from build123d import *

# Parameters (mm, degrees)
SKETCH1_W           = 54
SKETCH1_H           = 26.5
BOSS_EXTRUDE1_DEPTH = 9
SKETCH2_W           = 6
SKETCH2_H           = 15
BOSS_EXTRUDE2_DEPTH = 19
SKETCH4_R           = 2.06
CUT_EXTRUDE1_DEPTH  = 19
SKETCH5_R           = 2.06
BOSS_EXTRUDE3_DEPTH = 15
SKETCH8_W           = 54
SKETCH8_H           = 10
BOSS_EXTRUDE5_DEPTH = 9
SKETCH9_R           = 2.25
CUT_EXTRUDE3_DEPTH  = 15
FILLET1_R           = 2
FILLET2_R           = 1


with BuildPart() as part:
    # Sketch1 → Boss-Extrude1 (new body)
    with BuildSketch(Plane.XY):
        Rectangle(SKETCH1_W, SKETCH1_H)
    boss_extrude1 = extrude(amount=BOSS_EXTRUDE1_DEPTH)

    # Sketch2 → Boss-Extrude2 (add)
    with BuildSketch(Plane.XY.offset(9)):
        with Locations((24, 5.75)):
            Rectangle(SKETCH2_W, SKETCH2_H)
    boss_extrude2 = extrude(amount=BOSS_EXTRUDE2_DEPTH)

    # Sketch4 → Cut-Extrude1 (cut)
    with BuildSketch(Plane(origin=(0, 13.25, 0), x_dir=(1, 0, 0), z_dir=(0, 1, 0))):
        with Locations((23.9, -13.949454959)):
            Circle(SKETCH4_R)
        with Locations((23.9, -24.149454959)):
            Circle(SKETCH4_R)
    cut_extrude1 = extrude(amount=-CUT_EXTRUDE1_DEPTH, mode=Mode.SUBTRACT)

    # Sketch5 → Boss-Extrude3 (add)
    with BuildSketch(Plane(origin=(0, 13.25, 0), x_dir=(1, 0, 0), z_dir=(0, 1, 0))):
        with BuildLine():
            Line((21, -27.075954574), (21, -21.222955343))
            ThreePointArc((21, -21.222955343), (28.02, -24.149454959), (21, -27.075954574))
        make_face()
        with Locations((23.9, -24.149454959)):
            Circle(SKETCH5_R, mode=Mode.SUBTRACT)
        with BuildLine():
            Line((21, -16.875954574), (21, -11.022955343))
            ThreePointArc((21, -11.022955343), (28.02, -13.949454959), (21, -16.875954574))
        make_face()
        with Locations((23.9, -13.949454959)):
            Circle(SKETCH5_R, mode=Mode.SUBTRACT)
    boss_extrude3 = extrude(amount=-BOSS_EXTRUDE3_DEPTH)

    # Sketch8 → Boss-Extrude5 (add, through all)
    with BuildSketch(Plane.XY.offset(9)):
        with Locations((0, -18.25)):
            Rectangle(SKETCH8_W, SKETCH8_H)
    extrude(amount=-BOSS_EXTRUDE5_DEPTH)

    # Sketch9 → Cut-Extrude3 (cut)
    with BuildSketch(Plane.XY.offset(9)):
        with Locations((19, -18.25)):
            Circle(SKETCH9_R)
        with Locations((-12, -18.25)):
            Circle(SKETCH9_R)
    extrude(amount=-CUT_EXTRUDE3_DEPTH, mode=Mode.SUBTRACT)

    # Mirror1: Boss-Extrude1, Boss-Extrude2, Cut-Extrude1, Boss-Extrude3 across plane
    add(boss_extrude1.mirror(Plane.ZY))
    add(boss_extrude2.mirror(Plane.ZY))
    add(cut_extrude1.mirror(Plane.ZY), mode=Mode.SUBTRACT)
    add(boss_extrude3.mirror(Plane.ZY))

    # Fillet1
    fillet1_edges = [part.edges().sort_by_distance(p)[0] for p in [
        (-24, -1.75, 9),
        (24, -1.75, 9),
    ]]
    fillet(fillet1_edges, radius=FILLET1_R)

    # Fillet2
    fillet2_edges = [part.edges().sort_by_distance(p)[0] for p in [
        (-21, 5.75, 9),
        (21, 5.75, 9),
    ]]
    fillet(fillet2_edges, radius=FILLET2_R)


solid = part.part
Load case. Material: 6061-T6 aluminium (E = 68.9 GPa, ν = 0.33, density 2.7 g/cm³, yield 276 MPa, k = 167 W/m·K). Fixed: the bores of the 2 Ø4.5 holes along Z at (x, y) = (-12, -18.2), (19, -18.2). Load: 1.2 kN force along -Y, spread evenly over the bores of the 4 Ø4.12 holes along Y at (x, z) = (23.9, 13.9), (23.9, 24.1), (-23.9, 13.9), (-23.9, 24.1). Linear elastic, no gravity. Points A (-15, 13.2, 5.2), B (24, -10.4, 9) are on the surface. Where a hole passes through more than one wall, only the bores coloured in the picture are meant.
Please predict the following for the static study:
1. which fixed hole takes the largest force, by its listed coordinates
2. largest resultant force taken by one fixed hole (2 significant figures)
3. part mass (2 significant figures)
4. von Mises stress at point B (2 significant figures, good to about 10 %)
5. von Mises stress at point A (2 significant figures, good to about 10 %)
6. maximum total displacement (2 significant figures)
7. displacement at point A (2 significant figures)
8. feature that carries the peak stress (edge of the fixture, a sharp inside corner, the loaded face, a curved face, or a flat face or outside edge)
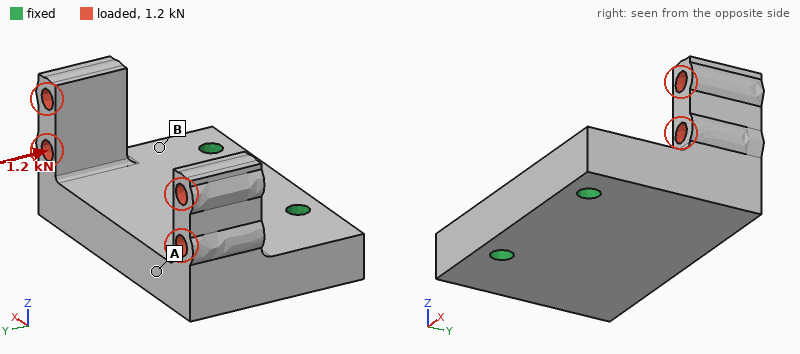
(-12, -18.2)
720 N
55 g
33 MPa
15 MPa
88 µm
43 µm
a curved face
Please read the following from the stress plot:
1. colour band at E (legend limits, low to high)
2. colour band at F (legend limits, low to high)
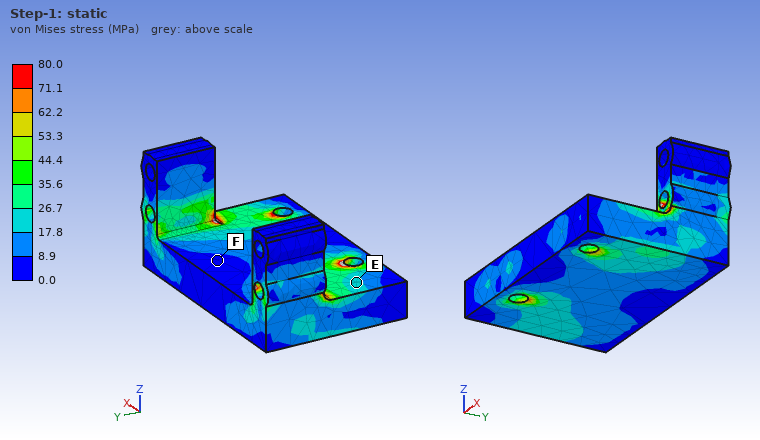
17.8 to 26.7 MPa
0.0 to 8.9 MPa
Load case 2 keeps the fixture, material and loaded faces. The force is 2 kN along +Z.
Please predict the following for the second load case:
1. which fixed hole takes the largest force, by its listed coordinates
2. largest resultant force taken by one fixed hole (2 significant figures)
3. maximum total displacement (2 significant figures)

(-12, -18.2)
1.1 kN
0.13 mm
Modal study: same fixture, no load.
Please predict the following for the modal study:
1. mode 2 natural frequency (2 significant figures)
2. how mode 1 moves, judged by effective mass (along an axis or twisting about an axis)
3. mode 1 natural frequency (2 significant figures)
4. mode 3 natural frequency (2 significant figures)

6200 Hz
along Z
4700 Hz
7800 Hz
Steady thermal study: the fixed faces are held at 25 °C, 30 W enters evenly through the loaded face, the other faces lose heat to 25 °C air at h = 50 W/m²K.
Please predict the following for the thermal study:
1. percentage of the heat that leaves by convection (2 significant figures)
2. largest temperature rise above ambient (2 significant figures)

11 %
27 K
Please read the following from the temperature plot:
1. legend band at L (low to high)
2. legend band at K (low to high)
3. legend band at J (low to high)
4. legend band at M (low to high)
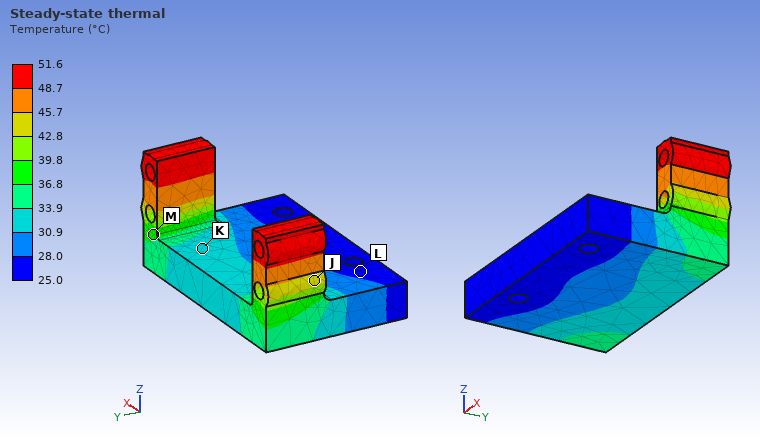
25.0 to 28.0 °C
30.9 to 33.9 °C
42.8 to 45.7 °C
36.8 to 39.8 °C
